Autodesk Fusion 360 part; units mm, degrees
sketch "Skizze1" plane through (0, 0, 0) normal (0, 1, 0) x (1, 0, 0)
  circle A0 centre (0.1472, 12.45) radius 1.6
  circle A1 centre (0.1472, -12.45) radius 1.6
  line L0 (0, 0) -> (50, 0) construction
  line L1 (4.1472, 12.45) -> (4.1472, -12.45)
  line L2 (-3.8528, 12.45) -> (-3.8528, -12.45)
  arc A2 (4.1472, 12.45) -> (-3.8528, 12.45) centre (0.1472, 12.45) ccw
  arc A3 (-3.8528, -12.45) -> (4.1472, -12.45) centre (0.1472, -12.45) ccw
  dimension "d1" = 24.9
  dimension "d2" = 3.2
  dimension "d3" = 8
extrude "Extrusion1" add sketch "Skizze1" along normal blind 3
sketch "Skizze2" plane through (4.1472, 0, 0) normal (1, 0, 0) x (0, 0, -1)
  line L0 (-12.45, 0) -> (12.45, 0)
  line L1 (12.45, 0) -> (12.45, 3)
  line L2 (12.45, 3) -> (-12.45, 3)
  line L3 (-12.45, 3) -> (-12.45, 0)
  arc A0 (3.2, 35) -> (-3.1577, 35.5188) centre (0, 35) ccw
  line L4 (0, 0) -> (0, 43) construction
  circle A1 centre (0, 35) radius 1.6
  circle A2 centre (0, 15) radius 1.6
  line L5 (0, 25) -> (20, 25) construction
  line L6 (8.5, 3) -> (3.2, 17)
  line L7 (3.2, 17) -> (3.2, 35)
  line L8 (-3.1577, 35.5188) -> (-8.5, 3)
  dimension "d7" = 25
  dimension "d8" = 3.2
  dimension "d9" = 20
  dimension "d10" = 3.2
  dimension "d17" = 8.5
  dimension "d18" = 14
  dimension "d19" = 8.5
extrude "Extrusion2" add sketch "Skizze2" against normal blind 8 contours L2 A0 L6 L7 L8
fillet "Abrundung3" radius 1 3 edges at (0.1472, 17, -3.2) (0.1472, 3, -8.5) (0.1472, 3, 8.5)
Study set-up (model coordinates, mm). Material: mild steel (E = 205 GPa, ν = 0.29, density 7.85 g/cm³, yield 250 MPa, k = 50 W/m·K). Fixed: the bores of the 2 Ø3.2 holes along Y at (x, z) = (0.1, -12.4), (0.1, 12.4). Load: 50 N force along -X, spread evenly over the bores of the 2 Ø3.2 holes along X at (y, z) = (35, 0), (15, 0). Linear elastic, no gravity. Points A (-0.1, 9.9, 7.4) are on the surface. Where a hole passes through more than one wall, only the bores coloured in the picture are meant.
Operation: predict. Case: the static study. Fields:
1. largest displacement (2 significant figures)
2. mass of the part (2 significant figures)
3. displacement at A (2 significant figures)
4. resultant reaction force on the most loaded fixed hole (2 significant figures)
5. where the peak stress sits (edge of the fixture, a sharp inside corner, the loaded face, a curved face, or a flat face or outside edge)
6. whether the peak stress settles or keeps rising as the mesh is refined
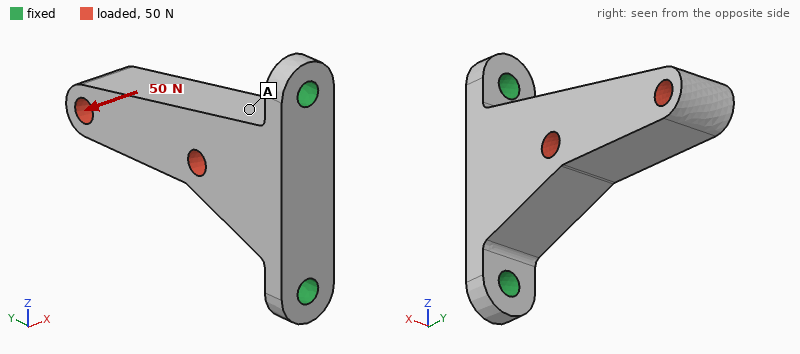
20 µm
26 g
3.9 µm
25 N
edge of the fixture
keeps rising
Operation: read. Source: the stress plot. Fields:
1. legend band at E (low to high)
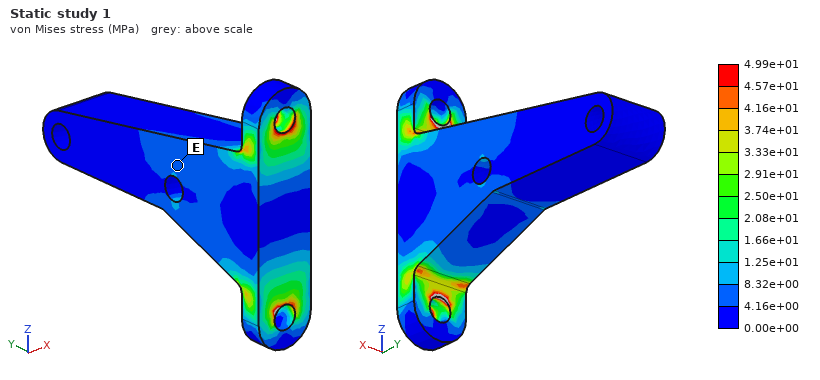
4.16e+00 to 8.32e+00 MPa
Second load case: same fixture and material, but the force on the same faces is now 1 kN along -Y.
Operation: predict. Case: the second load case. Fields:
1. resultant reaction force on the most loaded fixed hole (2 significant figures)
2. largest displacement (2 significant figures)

570 N
6.0 µm
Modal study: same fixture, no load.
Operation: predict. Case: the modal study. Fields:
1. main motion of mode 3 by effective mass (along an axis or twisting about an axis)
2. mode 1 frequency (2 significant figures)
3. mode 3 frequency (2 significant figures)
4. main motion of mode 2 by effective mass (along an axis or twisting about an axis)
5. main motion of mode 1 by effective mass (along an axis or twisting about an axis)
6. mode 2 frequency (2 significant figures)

along Y
2900 Hz
18 kHz
along Z
along X
8100 Hz
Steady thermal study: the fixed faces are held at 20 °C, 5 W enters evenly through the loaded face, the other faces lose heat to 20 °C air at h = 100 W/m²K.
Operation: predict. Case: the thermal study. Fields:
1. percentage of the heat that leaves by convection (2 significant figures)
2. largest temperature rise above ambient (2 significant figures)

43 %
27 K
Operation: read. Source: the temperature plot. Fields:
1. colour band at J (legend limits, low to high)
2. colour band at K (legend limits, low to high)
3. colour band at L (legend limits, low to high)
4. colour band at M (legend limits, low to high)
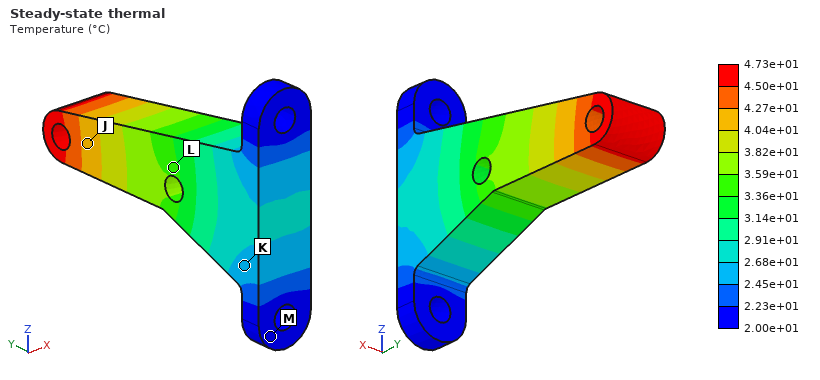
4.04e+01 to 4.27e+01 °C
2.45e+01 to 2.68e+01 °C
3.36e+01 to 3.59e+01 °C
2.00e+01 to 2.23e+01 °C
